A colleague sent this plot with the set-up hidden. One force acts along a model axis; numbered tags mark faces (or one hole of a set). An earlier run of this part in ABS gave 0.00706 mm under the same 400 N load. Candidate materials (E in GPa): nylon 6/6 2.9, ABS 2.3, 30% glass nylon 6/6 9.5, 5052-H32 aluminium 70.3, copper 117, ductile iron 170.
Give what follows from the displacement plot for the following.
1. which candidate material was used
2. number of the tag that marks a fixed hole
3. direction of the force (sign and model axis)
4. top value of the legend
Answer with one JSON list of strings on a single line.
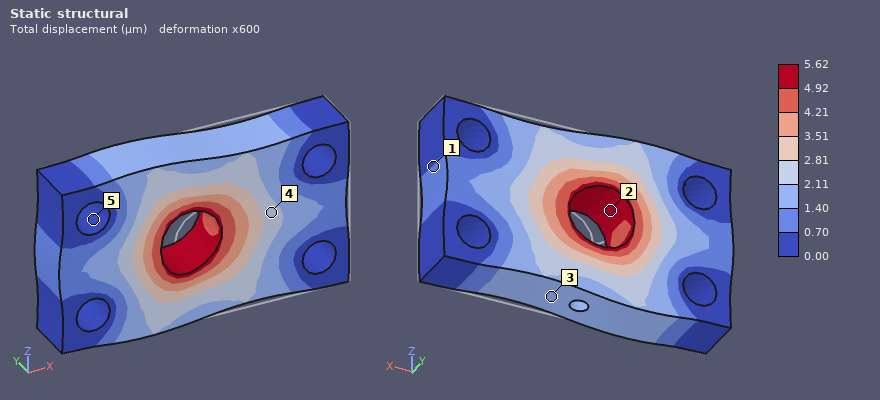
["nylon 6/6", "5", "-X", "5.62 µm"]
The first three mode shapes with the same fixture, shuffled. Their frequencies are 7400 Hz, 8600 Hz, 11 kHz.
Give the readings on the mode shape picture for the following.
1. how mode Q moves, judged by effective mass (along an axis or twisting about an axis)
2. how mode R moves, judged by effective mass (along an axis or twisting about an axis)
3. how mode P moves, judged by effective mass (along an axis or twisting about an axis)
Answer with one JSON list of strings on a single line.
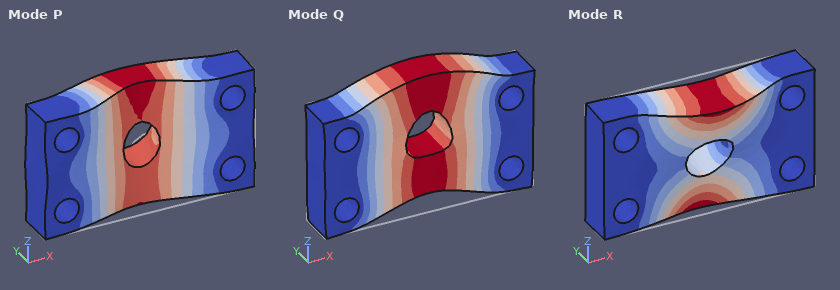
["along Z", "twisting about X", "along Y"]
